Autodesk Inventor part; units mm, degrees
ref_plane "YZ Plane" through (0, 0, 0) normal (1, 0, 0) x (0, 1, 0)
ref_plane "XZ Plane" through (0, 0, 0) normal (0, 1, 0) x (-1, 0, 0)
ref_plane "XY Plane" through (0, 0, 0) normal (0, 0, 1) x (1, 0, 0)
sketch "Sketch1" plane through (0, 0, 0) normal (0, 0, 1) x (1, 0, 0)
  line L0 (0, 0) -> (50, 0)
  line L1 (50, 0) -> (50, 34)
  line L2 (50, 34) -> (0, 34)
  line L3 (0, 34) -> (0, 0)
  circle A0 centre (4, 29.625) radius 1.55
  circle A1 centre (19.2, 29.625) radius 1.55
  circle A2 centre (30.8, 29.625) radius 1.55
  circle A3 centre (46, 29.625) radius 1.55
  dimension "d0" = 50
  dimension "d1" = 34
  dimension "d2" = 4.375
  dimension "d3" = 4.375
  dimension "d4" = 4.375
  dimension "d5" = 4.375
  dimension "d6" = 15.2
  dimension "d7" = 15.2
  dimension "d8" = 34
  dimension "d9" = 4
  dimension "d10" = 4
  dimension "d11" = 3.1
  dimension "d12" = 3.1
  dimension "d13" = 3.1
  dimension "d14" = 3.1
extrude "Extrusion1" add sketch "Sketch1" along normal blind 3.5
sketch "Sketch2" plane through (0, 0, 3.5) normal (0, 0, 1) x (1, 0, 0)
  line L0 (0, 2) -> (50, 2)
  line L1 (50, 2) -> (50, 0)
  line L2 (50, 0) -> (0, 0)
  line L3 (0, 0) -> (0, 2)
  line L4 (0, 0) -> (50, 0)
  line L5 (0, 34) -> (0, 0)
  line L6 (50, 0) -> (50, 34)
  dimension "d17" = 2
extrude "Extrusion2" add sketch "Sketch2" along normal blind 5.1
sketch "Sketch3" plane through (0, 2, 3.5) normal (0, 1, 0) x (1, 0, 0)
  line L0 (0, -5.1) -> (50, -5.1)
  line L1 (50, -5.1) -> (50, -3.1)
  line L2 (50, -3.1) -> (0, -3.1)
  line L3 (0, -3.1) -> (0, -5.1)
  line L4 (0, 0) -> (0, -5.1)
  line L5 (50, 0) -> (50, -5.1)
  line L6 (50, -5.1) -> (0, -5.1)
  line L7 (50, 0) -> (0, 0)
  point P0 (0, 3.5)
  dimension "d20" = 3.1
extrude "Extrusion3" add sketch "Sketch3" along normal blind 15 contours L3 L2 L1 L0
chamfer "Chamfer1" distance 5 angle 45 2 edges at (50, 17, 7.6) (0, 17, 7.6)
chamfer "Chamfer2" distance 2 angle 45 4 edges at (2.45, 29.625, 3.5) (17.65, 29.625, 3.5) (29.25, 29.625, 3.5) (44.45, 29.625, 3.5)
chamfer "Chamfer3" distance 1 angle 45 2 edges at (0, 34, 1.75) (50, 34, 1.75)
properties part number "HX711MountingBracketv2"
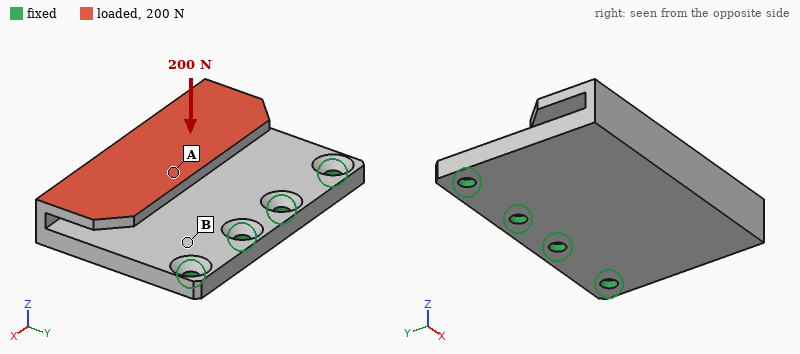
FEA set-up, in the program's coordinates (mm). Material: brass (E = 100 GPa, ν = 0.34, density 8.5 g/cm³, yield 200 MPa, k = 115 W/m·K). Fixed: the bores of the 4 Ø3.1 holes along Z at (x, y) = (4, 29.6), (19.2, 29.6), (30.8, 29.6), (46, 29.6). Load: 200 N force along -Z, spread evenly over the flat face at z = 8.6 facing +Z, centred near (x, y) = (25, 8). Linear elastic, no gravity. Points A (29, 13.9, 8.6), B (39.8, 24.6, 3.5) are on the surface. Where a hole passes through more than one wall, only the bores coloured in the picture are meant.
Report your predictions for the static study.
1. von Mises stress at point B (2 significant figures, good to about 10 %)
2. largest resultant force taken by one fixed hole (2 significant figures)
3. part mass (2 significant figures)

32 MPa
66 N
65 g
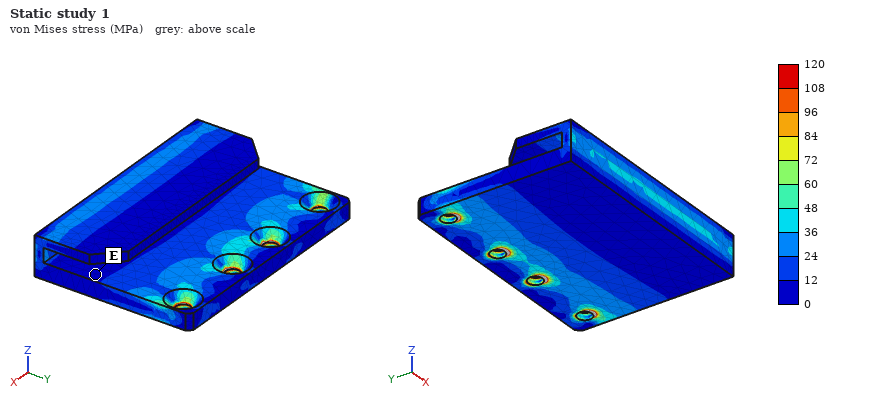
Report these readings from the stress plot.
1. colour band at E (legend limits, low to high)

0 to 12 MPa
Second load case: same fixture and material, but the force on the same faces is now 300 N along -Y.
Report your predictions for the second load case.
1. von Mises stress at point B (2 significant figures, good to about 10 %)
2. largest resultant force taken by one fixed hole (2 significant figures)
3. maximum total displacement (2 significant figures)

21 MPa
80 N
78 µm
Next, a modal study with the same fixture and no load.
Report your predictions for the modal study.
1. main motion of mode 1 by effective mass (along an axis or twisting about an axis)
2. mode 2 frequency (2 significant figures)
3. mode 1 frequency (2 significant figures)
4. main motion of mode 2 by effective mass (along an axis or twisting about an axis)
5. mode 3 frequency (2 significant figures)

along Z
2300 Hz
1300 Hz
twisting about Y
3100 Hz
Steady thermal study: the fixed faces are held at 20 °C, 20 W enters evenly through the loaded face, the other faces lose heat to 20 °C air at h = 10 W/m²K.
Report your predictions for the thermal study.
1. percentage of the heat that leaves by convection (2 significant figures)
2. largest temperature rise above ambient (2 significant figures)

5.4 %
49 K
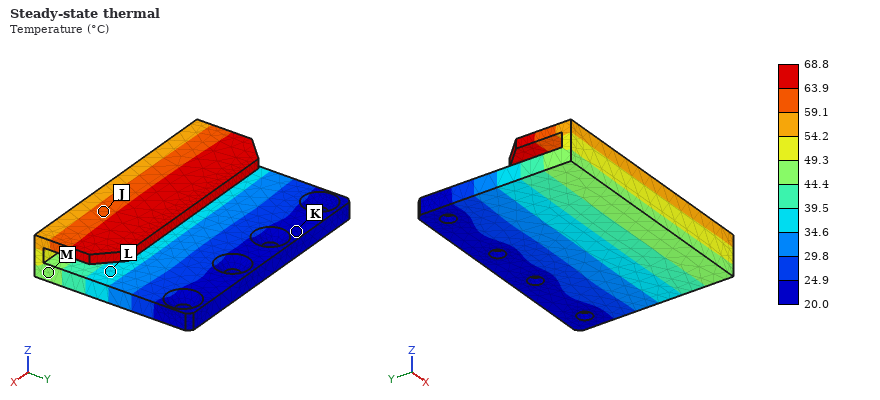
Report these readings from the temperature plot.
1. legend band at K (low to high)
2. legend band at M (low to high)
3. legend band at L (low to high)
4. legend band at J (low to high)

20.0 to 24.9 °C
44.4 to 49.3 °C
34.6 to 39.5 °C
59.1 to 63.9 °C
